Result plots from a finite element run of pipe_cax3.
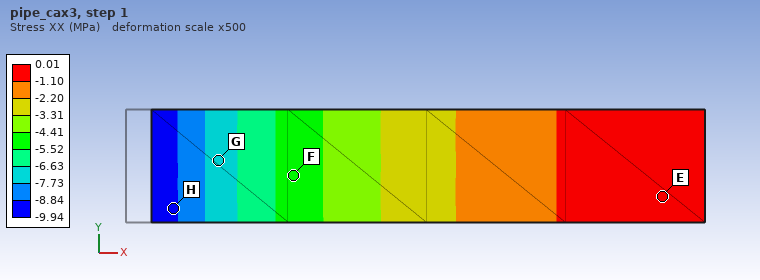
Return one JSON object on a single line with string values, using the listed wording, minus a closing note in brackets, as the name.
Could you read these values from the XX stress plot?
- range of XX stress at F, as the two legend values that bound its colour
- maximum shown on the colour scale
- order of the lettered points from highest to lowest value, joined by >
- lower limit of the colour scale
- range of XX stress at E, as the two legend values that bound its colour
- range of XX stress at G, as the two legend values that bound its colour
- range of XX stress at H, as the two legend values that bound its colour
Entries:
{"range of XX stress at F, as the two legend values that bound its colour": "-5.52 to -4.41 MPa", "maximum shown on the colour scale": "0.01 MPa", "order of the lettered points from highest to lowest value, joined by >": "E > F > G > H", "lower limit of the colour scale": "-9.94 MPa", "range of XX stress at E, as the two legend values that bound its colour": "-1.10 to 0.01 MPa", "range of XX stress at G, as the two legend values that bound its colour": "-7.73 to -6.63 MPa", "range of XX stress at H, as the two legend values that bound its colour": "-9.94 to -8.84 MPa"}
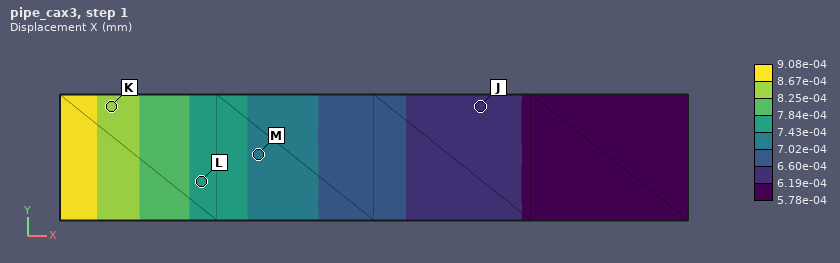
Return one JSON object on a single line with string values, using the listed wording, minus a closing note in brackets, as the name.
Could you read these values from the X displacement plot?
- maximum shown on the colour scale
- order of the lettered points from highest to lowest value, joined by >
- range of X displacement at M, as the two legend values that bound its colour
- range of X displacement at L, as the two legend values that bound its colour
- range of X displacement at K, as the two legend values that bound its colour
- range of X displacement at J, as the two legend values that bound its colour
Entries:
{"maximum shown on the colour scale": "9.08e-04 mm", "order of the lettered points from highest to lowest value, joined by >": "K > L > M > J", "range of X displacement at M, as the two legend values that bound its colour": "7.02e-04 to 7.43e-04 mm", "range of X displacement at L, as the two legend values that bound its colour": "7.43e-04 to 7.84e-04 mm", "range of X displacement at K, as the two legend values that bound its colour": "8.25e-04 to 8.67e-04 mm", "range of X displacement at J, as the two legend values that bound its colour": "6.19e-04 to 6.60e-04 mm"}
